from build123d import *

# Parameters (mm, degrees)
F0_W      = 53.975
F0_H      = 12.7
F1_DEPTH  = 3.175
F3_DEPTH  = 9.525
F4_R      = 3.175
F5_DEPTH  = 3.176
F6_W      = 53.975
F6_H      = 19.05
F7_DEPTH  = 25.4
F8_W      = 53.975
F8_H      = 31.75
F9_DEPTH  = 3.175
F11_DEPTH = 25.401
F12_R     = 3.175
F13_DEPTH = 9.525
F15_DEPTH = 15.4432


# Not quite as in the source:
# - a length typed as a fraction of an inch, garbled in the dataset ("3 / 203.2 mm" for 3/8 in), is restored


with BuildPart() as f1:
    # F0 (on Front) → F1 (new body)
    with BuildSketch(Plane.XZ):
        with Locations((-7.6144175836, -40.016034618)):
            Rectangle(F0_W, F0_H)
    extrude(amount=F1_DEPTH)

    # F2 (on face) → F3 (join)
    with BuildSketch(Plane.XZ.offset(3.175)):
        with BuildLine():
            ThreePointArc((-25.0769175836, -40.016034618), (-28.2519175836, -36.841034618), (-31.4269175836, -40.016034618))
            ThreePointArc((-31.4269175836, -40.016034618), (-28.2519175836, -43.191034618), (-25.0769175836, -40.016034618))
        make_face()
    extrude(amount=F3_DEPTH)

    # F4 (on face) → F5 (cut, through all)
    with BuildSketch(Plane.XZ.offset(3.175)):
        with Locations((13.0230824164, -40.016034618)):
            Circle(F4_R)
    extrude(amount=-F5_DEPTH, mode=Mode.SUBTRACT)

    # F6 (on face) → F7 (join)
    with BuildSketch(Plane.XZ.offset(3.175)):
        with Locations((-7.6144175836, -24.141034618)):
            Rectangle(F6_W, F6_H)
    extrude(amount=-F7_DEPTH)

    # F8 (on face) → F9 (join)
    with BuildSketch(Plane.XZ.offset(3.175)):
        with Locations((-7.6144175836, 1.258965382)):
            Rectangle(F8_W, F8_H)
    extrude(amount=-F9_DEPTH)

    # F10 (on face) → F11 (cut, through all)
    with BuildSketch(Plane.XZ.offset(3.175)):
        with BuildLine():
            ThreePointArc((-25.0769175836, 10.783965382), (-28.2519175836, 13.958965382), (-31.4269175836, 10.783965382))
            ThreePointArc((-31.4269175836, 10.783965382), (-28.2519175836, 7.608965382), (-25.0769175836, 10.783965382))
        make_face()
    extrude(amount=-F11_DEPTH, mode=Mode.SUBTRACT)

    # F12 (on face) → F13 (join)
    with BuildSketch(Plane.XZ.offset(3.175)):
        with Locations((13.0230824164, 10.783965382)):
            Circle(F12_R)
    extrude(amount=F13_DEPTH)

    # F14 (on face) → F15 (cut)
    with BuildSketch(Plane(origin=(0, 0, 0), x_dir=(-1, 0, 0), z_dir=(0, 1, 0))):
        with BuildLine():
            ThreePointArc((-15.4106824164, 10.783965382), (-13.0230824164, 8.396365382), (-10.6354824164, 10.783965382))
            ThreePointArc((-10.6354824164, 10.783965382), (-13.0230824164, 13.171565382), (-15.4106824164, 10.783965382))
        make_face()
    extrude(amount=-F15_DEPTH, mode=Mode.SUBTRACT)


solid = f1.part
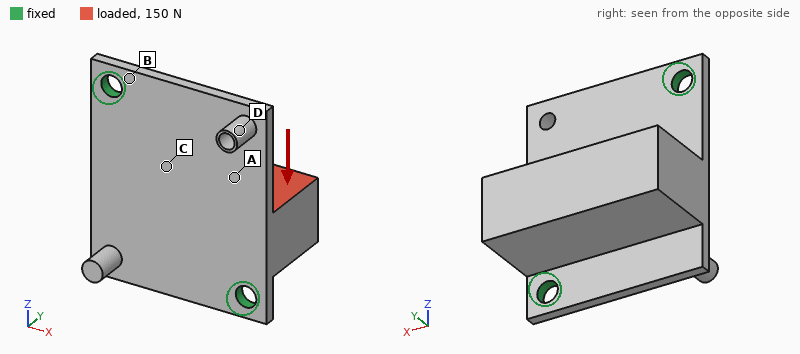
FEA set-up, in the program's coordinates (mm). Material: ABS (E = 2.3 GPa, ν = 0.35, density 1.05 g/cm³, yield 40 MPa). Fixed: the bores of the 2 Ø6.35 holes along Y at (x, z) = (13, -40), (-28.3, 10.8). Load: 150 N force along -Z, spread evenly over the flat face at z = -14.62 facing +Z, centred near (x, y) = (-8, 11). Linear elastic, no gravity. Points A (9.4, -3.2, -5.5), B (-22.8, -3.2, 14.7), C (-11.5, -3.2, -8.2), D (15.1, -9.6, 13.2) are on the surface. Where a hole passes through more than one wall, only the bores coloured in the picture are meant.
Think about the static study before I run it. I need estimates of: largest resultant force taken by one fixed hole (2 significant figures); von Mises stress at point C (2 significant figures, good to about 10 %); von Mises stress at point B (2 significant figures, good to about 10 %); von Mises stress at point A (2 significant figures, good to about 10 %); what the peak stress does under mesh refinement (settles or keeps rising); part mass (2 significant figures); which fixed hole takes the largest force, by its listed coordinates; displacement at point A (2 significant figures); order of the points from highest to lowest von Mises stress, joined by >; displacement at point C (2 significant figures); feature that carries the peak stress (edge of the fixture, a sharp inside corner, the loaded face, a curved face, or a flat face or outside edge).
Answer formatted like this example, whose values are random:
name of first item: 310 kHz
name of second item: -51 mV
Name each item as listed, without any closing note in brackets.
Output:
largest resultant force taken by one fixed hole: 93 N
von Mises stress at point C: 4.8 MPa
von Mises stress at point B: 7.3 MPa
von Mises stress at point A: 3.7 MPa
what the peak stress does under mesh refinement: keeps rising
part mass: 36 g
which fixed hole takes the largest force, by its listed coordinates: (13, -40)
displacement at point A: 0.57 mm
order of the points from highest to lowest von Mises stress, joined by >: B > C > A > D
displacement at point C: 0.21 mm
feature that carries the peak stress: edge of the fixture
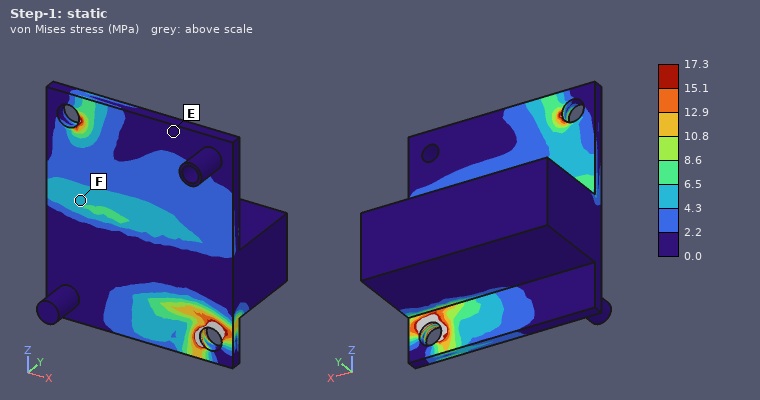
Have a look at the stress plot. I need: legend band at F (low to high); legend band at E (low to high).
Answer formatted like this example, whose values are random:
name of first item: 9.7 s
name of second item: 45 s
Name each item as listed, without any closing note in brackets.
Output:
legend band at F: 4.3 to 6.5 MPa
legend band at E: 0.0 to 2.2 MPa
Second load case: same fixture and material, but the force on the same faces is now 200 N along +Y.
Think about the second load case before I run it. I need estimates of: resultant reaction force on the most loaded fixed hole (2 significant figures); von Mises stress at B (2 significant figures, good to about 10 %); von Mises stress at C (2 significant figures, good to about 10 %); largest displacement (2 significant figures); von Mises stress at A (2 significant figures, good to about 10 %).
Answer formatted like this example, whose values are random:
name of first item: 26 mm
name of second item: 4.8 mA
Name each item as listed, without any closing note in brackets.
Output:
resultant reaction force on the most loaded fixed hole: 110 N
von Mises stress at B: 8.7 MPa
von Mises stress at C: 11 MPa
largest displacement: 0.87 mm
von Mises stress at A: 5.7 MPa
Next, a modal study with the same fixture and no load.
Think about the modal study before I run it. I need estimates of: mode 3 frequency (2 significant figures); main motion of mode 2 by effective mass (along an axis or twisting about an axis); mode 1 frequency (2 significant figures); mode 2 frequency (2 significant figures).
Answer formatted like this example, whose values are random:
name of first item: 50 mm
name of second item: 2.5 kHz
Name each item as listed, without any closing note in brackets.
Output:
mode 3 frequency: 1100 Hz
main motion of mode 2 by effective mass: along Y
mode 1 frequency: 340 Hz
mode 2 frequency: 590 Hz
